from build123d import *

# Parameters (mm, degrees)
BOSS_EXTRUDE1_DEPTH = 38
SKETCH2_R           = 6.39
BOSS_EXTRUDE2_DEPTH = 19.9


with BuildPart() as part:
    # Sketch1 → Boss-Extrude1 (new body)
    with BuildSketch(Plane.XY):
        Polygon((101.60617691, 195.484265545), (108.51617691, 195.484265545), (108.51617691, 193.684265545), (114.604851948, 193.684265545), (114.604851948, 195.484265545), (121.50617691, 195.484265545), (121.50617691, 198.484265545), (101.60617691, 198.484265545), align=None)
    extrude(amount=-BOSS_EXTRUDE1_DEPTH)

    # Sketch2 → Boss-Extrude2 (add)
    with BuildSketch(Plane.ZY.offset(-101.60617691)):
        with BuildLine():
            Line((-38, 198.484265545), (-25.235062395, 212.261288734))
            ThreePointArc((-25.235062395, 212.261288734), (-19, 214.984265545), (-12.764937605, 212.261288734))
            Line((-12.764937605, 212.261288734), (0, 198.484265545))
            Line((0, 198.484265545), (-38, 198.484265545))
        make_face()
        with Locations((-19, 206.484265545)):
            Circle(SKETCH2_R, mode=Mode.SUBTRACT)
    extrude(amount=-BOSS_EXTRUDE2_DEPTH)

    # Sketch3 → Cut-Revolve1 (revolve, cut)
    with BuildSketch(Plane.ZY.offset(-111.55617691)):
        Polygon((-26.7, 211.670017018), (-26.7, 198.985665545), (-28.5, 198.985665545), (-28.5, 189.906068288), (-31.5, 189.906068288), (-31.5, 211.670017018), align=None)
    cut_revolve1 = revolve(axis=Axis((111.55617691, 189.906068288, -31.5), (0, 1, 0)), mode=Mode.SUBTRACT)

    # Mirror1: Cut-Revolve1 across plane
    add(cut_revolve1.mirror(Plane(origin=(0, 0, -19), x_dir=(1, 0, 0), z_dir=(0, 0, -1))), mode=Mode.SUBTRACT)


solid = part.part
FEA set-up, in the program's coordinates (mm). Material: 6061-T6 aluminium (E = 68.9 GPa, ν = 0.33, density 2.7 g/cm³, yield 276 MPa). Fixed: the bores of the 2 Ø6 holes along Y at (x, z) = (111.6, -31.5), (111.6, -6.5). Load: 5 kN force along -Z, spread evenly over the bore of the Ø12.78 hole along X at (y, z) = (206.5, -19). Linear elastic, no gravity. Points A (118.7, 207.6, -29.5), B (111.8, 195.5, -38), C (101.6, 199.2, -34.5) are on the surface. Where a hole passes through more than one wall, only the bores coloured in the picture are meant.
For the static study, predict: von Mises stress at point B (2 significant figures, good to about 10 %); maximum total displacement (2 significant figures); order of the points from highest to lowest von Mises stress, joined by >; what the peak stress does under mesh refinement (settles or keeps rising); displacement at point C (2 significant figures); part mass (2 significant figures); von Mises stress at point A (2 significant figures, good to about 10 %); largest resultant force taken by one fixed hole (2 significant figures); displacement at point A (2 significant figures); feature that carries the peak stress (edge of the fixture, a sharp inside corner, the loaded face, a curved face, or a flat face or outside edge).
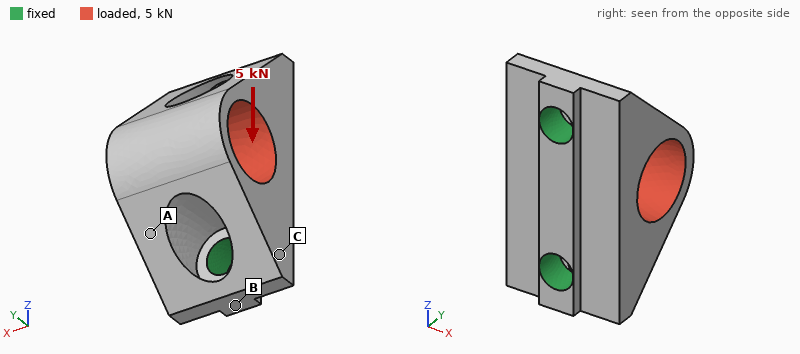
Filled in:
36 MPa
37 µm
A > B > C
keeps rising
11 µm
17 g
72 MPa
3.0 kN
19 µm
edge of the fixture
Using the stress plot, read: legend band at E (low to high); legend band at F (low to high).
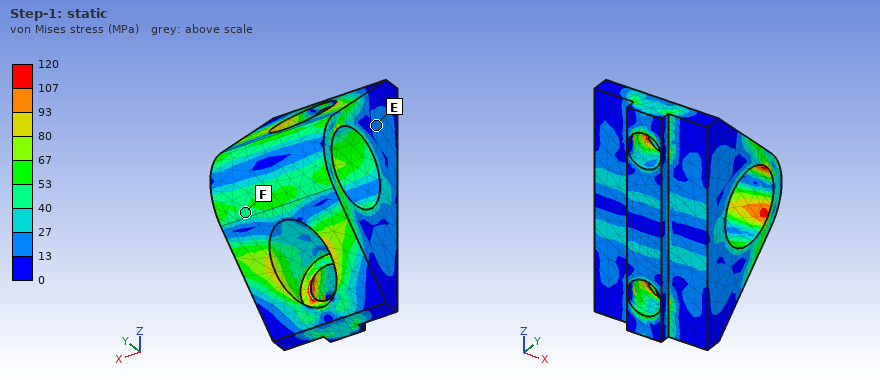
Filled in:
13 to 27 MPa
40 to 53 MPa
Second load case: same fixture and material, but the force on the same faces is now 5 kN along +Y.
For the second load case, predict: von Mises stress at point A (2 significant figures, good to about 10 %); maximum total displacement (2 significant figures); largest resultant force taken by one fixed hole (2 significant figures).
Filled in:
28 MPa
15 µm
2.6 kN
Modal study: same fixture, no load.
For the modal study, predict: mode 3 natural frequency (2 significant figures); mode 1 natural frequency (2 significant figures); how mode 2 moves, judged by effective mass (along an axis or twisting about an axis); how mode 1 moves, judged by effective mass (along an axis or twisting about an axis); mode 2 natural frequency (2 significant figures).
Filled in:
30 kHz
14 kHz
along Z
along X
26 kHz
